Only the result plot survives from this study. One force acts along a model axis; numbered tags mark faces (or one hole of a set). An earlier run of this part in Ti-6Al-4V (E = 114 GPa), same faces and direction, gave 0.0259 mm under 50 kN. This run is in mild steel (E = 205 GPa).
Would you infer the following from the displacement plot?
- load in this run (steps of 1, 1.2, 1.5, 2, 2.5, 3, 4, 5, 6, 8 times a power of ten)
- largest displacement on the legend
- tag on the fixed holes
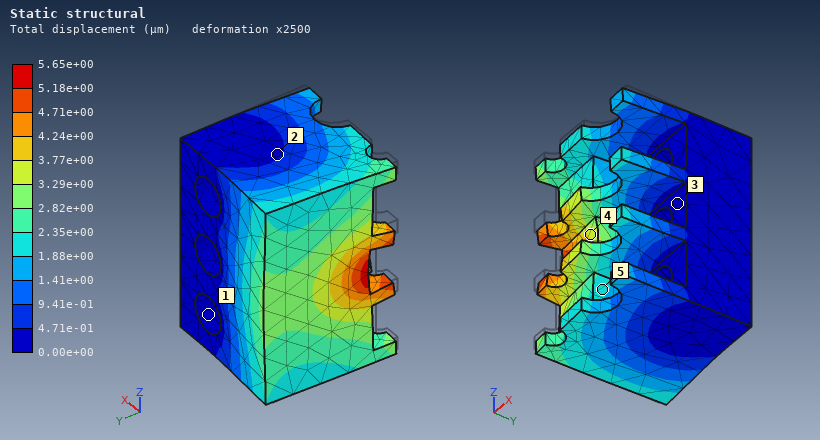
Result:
20 kN
5.65e+00 µm
1
